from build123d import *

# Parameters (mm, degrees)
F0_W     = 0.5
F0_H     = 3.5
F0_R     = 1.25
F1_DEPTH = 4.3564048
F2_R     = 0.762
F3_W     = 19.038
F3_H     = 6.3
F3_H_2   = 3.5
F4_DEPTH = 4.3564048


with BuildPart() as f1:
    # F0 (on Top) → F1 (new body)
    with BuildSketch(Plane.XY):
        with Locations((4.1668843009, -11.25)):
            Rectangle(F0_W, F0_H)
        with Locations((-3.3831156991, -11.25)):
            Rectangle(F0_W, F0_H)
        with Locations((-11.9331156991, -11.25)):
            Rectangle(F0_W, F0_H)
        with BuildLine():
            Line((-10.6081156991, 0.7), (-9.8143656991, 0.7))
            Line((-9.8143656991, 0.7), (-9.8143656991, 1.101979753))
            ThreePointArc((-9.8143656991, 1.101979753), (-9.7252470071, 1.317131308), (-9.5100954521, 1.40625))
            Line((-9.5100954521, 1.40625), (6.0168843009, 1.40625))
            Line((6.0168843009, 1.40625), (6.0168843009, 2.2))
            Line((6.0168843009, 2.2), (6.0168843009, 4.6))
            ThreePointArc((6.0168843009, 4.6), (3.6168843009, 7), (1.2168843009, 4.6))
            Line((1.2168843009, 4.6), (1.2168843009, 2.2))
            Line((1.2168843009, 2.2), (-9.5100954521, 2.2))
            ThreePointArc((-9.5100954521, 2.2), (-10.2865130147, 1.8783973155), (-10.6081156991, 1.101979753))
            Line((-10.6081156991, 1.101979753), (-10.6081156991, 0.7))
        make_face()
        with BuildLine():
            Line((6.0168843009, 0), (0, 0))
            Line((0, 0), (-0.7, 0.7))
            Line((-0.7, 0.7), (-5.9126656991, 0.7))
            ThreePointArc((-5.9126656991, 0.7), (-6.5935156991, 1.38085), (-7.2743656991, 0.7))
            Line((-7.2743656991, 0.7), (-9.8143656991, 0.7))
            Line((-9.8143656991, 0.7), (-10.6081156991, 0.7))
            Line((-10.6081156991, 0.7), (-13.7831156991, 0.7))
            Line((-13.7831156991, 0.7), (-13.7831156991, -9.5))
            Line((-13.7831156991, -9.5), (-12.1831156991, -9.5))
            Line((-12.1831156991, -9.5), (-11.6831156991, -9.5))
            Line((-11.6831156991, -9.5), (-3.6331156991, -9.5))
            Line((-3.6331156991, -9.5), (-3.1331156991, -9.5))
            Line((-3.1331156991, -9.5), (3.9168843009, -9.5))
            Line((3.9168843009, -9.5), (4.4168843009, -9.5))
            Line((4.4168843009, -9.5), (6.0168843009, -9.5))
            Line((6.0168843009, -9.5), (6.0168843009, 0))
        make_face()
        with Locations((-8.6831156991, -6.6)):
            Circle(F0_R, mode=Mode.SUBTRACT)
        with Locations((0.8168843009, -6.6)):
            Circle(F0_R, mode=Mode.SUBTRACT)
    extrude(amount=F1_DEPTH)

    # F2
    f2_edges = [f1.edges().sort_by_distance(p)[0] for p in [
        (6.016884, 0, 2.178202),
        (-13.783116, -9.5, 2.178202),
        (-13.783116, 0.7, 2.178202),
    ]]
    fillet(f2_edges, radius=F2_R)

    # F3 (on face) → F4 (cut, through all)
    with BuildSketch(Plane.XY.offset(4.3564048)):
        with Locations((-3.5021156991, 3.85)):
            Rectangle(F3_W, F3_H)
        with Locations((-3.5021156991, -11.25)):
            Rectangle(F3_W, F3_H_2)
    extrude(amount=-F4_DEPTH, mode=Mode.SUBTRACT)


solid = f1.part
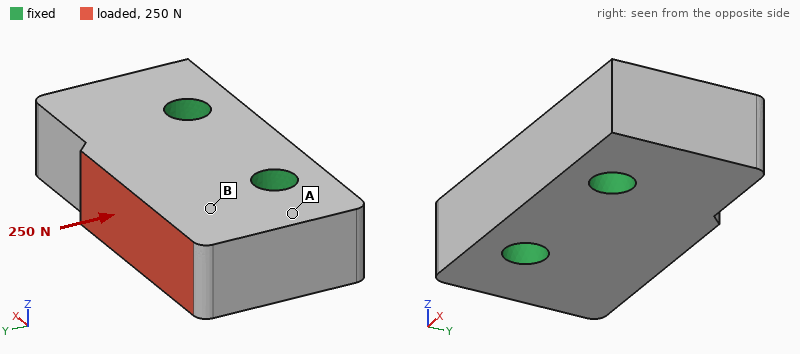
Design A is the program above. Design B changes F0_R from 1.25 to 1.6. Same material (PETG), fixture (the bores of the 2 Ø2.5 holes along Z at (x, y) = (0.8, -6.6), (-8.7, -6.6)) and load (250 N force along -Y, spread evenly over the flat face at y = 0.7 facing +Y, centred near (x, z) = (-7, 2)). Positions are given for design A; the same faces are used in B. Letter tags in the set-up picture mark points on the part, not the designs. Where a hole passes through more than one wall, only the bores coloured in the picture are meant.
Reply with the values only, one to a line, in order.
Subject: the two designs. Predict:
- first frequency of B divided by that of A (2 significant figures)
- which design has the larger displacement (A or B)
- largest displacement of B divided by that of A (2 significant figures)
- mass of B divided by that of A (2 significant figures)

1.1
A
0.87
0.97
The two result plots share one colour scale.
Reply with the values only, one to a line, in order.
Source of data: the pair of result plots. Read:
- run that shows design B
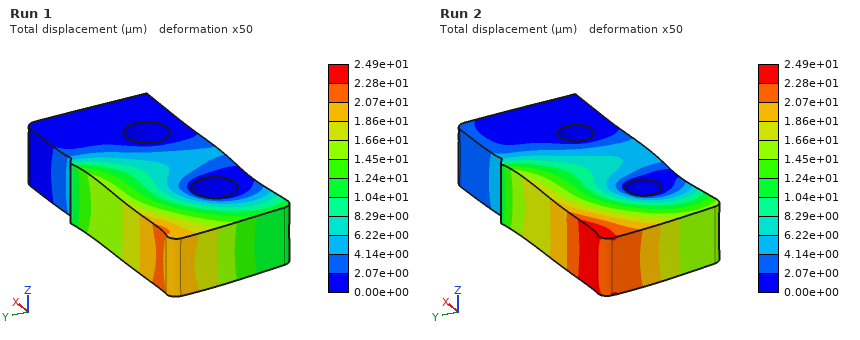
Run 1
